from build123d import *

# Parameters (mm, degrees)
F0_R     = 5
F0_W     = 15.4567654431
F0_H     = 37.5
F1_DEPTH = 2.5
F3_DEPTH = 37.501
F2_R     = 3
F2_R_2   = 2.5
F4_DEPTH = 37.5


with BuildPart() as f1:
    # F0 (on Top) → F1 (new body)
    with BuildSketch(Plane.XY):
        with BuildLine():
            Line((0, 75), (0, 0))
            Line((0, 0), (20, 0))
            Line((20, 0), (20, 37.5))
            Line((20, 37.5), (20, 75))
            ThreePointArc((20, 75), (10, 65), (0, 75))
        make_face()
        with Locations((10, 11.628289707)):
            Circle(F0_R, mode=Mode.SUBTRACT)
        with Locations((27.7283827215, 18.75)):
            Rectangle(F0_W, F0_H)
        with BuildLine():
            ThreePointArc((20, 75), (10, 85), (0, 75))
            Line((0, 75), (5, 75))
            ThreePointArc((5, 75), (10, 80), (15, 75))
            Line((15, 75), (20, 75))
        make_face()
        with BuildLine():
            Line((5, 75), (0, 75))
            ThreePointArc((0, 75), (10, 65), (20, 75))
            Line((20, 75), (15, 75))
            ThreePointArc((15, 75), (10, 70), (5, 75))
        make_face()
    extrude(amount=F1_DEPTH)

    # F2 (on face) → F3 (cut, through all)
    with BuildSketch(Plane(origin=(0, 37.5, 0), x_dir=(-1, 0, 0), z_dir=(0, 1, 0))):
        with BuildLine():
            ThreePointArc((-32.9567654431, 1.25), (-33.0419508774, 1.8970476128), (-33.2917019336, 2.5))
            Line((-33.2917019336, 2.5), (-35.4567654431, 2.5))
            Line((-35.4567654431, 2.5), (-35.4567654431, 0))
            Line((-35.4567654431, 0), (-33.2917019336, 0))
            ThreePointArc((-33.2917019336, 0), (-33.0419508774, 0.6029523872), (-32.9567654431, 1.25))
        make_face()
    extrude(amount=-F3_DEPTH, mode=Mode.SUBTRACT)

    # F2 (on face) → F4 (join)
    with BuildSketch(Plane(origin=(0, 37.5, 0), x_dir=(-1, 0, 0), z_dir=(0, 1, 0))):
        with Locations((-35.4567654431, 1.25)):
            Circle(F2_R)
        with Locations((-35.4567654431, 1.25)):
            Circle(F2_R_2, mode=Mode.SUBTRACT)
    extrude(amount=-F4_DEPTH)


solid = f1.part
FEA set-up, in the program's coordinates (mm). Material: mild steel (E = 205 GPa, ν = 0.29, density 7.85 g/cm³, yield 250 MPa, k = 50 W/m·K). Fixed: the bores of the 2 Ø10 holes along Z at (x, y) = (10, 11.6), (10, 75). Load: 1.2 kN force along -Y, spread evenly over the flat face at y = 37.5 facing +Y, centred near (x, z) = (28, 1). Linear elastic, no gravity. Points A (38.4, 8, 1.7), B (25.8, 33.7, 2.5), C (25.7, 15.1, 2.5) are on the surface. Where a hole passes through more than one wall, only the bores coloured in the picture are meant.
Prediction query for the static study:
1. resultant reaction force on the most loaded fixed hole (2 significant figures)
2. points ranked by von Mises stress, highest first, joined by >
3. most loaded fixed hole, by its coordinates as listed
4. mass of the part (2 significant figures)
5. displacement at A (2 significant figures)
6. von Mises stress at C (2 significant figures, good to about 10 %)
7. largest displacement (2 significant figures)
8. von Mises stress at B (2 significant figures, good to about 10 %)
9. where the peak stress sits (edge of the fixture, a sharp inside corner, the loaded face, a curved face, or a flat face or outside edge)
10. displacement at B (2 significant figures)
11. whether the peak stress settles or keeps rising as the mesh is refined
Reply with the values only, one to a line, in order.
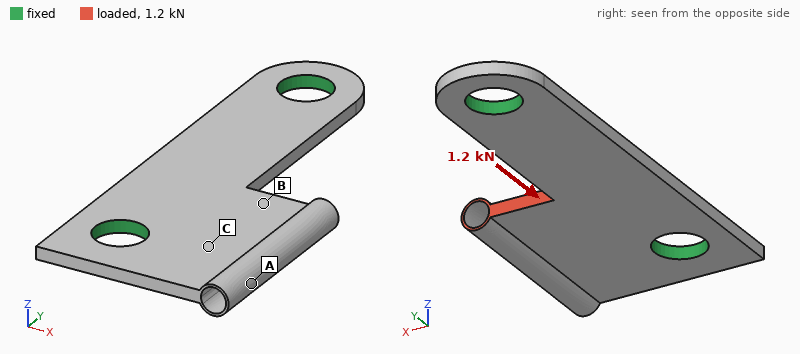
980 N
B > C > A
(10, 11.6)
41 g
7.3 µm
19 MPa
12 µm
33 MPa
a sharp inside corner
6.7 µm
keeps rising
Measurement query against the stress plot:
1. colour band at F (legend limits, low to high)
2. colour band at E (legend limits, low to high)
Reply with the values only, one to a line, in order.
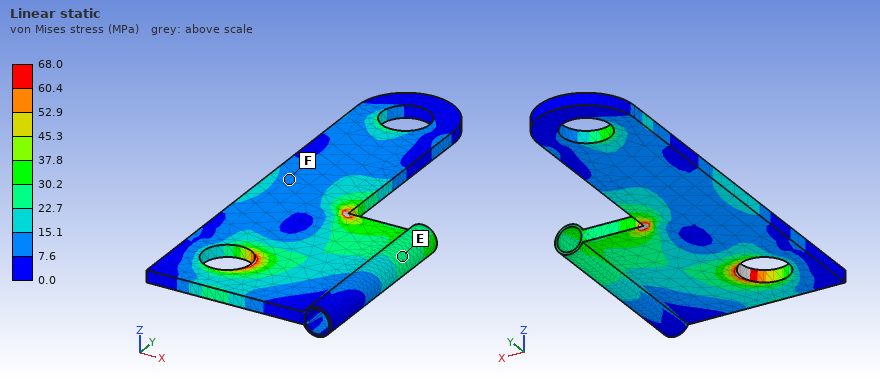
7.6 to 15.1 MPa
22.7 to 30.2 MPa
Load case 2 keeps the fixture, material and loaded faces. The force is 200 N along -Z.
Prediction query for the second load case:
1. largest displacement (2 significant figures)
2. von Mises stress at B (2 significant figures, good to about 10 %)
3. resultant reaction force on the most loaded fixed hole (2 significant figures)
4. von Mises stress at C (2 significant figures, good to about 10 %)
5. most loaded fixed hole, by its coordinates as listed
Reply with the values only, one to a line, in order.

0.15 mm
64 MPa
150 N
54 MPa
(10, 11.6)
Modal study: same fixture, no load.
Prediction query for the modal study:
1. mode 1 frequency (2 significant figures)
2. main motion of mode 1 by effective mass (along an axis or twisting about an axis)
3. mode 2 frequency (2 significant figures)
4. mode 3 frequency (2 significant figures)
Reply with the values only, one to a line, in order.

3100 Hz
along Z
4300 Hz
6100 Hz
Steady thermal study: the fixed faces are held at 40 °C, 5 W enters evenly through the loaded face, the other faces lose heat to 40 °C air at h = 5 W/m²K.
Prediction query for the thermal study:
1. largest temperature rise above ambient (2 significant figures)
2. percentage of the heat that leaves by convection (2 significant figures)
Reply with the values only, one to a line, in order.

48 K
6.0 %
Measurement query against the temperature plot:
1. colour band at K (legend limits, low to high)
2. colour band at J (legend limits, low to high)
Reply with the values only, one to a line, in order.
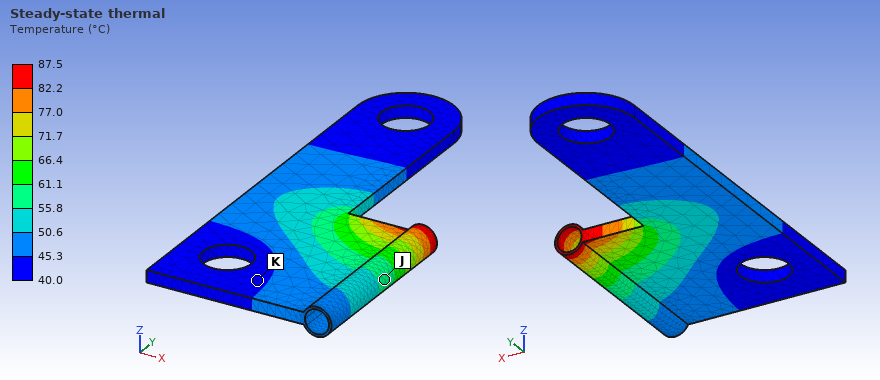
40.0 to 45.3 °C
55.8 to 61.1 °C
